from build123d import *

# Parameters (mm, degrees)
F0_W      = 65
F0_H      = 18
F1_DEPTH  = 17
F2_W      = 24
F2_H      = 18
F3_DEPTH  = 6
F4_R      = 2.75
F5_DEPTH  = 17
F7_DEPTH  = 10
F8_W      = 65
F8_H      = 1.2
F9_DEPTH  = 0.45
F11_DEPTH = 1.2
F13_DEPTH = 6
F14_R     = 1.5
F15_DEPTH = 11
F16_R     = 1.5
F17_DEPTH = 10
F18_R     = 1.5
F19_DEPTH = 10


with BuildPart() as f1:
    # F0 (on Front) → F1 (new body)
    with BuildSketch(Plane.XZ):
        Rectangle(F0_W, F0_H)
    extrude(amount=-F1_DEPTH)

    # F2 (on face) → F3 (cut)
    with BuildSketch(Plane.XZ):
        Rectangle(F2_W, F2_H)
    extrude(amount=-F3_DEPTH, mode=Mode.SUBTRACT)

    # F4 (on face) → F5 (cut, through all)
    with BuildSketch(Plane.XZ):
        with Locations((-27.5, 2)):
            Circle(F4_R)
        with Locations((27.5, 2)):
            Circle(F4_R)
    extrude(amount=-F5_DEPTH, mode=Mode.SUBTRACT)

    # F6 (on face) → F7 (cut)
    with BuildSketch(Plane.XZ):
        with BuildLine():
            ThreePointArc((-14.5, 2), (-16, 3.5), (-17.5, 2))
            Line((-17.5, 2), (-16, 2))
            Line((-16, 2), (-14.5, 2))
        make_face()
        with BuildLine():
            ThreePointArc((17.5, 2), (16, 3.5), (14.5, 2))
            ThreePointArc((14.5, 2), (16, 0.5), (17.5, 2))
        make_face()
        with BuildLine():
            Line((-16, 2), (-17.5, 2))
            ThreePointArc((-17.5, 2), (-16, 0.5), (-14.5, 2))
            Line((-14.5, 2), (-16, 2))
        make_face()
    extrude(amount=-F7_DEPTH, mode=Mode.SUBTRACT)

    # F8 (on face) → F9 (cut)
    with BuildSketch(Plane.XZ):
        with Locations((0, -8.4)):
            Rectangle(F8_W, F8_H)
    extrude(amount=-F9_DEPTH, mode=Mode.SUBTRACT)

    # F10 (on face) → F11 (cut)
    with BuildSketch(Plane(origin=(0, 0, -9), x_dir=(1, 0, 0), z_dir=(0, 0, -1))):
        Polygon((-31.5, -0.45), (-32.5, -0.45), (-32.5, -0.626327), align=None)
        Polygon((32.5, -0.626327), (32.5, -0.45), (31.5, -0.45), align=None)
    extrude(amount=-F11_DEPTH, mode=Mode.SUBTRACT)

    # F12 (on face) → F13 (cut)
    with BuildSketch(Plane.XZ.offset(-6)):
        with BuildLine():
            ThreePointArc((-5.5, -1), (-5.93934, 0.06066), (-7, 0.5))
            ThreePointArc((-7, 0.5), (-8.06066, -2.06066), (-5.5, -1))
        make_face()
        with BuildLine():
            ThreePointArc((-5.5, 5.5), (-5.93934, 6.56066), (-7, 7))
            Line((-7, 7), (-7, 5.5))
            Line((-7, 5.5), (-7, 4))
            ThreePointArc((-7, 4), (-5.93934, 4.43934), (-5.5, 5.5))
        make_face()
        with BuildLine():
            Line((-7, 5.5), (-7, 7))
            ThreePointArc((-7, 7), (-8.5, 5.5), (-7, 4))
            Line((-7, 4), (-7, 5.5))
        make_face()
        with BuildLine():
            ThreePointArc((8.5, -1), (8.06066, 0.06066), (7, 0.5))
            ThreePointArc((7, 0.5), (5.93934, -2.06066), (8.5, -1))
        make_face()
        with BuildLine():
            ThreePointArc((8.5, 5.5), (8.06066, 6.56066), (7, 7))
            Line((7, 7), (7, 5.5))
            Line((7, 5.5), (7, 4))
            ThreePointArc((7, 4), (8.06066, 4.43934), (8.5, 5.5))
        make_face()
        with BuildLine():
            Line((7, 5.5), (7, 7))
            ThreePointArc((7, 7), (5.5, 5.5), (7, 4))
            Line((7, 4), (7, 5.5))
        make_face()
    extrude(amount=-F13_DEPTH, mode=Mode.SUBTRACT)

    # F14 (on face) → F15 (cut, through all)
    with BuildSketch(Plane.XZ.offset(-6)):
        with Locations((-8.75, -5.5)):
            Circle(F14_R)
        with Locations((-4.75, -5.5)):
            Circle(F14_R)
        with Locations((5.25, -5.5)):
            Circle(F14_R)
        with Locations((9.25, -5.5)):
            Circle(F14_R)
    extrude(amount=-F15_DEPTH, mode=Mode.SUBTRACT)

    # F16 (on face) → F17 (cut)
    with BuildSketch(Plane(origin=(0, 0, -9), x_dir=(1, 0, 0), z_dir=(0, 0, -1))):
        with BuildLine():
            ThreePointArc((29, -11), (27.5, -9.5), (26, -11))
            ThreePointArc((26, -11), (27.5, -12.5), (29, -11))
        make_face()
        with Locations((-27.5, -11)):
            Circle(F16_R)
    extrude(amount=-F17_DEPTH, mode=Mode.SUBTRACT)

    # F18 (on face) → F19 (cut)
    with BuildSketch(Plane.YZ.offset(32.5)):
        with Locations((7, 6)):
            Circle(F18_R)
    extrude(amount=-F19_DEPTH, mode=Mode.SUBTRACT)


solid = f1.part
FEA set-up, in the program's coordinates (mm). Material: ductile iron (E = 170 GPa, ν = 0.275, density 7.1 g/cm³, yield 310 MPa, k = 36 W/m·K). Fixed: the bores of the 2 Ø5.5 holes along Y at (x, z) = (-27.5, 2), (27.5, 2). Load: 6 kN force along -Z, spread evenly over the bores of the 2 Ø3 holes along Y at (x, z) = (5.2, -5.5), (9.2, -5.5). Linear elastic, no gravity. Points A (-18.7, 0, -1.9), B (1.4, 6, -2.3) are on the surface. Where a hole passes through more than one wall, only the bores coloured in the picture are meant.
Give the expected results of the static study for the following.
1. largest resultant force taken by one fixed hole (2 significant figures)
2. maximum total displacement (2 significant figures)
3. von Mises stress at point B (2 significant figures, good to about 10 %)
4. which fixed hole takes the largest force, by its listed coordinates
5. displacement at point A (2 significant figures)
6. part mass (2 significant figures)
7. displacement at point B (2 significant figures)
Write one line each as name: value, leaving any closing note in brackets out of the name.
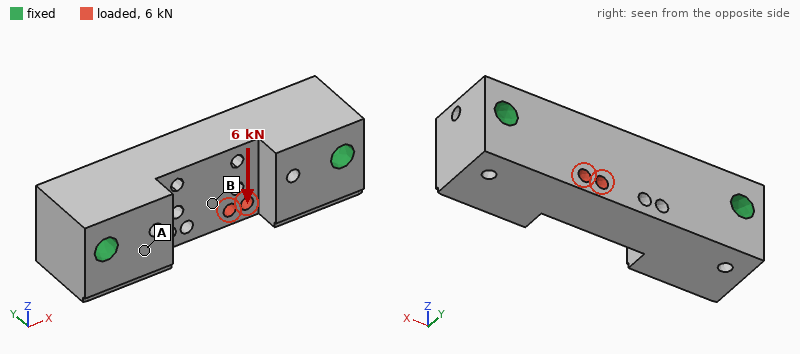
largest resultant force taken by one fixed hole: 4.1 kN
maximum total displacement: 16 µm
von Mises stress at point B: 30 MPa
which fixed hole takes the largest force, by its listed coordinates: (27.5, 2)
displacement at point A: 2.6 µm
part mass: 110 g
displacement at point B: 13 µm
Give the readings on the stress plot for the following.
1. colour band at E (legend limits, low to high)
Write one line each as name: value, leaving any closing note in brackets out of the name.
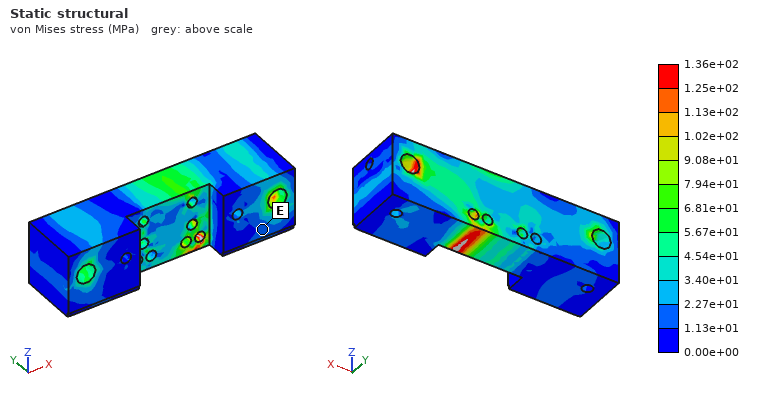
colour band at E: 1.13e+01 to 2.27e+01 MPa
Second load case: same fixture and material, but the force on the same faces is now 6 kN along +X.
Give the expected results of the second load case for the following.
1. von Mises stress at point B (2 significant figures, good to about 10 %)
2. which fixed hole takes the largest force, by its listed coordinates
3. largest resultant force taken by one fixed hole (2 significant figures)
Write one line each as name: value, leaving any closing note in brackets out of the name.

von Mises stress at point B: 25 MPa
which fixed hole takes the largest force, by its listed coordinates: (27.5, 2)
largest resultant force taken by one fixed hole: 3.8 kN
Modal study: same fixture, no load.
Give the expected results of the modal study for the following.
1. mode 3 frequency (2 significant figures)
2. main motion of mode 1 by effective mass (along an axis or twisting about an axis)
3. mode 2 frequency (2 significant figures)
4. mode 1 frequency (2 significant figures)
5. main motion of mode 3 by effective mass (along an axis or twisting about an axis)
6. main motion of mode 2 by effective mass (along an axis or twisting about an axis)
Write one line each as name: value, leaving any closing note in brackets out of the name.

mode 3 frequency: 30 kHz
main motion of mode 1 by effective mass: along Z
mode 2 frequency: 20 kHz
mode 1 frequency: 17 kHz
main motion of mode 3 by effective mass: twisting about X
main motion of mode 2 by effective mass: along Y
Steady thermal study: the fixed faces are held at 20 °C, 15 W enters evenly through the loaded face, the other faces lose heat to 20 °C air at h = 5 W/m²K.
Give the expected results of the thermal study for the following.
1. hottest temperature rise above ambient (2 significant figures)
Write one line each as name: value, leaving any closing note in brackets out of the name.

hottest temperature rise above ambient: 34 K
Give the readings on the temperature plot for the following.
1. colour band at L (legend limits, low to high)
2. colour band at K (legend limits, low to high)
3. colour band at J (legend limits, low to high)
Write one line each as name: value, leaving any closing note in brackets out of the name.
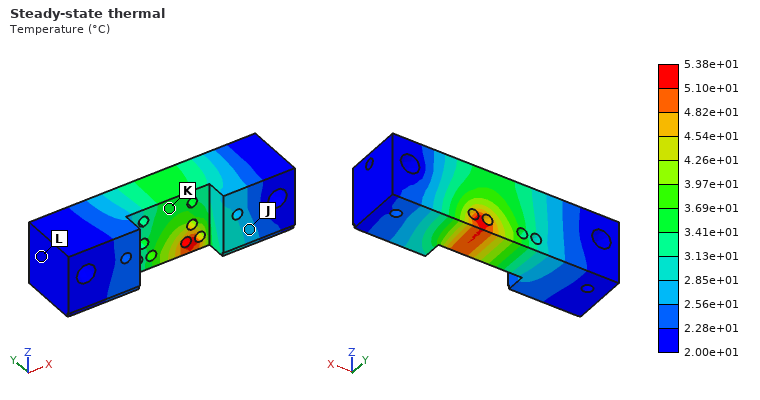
colour band at L: 2.00e+01 to 2.28e+01 °C
colour band at K: 3.41e+01 to 3.69e+01 °C
colour band at J: 2.56e+01 to 2.85e+01 °C
